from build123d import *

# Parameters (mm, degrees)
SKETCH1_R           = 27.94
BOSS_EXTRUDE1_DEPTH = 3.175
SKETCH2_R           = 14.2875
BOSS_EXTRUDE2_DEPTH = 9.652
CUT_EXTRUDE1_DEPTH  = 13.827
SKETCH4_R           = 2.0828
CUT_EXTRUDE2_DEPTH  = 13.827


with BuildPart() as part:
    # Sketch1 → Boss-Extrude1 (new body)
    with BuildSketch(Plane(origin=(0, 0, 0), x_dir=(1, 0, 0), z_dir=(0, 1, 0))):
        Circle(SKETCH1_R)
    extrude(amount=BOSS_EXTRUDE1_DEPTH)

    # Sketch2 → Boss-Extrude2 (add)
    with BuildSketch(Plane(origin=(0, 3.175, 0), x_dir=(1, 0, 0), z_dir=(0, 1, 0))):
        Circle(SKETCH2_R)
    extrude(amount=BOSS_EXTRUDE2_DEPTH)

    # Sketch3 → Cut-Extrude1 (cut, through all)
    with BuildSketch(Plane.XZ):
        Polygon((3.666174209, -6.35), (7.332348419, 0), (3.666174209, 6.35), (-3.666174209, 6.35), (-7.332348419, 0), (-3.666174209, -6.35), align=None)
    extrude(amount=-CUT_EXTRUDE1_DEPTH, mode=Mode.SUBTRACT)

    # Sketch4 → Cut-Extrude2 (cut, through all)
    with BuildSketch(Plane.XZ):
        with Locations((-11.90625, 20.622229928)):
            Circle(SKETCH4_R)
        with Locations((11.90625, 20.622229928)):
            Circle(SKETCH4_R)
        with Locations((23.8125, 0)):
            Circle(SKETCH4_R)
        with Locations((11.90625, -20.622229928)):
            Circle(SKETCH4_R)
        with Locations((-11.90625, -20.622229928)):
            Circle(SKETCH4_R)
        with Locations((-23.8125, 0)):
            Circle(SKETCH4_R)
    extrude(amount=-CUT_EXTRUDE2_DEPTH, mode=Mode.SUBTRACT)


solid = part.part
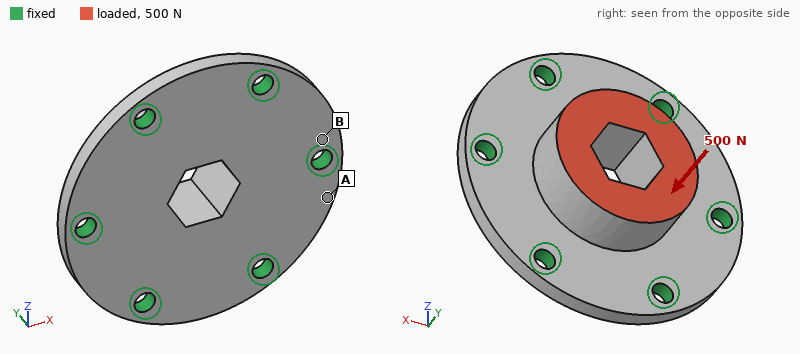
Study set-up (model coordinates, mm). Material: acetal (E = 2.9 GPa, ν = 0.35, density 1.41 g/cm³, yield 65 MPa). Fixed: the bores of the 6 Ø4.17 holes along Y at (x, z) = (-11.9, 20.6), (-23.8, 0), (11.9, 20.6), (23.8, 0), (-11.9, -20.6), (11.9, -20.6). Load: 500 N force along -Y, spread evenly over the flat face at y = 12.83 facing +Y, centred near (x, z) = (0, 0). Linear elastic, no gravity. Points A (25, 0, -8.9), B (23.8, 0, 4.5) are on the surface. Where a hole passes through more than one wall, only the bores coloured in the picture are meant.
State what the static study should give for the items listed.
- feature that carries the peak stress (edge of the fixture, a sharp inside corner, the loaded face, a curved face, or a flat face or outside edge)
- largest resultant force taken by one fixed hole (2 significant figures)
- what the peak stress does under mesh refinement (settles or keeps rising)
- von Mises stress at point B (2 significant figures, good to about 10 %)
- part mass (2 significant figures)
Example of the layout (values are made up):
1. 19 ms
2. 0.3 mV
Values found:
1. edge of the fixture
2. 94 N
3. keeps rising
4. 5.1 MPa
5. 17 g
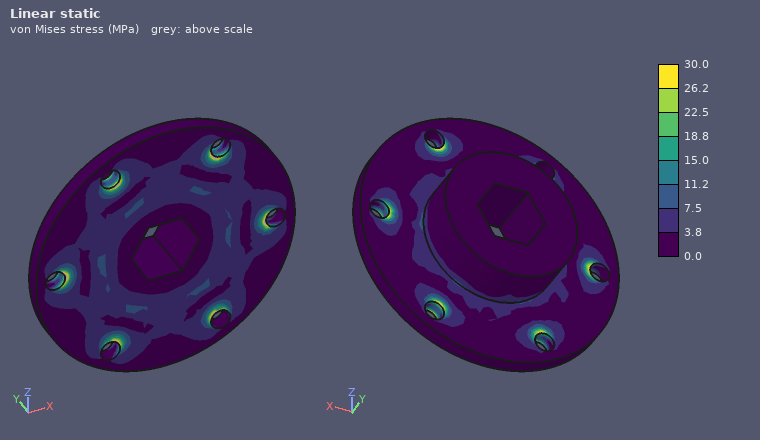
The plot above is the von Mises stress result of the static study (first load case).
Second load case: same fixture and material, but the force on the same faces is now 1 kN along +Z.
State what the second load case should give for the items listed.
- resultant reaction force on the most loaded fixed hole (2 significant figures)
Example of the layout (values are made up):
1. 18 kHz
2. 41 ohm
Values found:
1. 270 N
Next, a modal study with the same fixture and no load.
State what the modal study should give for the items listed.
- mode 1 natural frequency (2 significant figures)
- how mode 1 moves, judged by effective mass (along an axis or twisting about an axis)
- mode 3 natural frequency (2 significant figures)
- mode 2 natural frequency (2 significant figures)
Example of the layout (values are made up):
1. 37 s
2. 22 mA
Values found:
1. 3700 Hz
2. along Y
3. 4900 Hz
4. 4900 Hz
